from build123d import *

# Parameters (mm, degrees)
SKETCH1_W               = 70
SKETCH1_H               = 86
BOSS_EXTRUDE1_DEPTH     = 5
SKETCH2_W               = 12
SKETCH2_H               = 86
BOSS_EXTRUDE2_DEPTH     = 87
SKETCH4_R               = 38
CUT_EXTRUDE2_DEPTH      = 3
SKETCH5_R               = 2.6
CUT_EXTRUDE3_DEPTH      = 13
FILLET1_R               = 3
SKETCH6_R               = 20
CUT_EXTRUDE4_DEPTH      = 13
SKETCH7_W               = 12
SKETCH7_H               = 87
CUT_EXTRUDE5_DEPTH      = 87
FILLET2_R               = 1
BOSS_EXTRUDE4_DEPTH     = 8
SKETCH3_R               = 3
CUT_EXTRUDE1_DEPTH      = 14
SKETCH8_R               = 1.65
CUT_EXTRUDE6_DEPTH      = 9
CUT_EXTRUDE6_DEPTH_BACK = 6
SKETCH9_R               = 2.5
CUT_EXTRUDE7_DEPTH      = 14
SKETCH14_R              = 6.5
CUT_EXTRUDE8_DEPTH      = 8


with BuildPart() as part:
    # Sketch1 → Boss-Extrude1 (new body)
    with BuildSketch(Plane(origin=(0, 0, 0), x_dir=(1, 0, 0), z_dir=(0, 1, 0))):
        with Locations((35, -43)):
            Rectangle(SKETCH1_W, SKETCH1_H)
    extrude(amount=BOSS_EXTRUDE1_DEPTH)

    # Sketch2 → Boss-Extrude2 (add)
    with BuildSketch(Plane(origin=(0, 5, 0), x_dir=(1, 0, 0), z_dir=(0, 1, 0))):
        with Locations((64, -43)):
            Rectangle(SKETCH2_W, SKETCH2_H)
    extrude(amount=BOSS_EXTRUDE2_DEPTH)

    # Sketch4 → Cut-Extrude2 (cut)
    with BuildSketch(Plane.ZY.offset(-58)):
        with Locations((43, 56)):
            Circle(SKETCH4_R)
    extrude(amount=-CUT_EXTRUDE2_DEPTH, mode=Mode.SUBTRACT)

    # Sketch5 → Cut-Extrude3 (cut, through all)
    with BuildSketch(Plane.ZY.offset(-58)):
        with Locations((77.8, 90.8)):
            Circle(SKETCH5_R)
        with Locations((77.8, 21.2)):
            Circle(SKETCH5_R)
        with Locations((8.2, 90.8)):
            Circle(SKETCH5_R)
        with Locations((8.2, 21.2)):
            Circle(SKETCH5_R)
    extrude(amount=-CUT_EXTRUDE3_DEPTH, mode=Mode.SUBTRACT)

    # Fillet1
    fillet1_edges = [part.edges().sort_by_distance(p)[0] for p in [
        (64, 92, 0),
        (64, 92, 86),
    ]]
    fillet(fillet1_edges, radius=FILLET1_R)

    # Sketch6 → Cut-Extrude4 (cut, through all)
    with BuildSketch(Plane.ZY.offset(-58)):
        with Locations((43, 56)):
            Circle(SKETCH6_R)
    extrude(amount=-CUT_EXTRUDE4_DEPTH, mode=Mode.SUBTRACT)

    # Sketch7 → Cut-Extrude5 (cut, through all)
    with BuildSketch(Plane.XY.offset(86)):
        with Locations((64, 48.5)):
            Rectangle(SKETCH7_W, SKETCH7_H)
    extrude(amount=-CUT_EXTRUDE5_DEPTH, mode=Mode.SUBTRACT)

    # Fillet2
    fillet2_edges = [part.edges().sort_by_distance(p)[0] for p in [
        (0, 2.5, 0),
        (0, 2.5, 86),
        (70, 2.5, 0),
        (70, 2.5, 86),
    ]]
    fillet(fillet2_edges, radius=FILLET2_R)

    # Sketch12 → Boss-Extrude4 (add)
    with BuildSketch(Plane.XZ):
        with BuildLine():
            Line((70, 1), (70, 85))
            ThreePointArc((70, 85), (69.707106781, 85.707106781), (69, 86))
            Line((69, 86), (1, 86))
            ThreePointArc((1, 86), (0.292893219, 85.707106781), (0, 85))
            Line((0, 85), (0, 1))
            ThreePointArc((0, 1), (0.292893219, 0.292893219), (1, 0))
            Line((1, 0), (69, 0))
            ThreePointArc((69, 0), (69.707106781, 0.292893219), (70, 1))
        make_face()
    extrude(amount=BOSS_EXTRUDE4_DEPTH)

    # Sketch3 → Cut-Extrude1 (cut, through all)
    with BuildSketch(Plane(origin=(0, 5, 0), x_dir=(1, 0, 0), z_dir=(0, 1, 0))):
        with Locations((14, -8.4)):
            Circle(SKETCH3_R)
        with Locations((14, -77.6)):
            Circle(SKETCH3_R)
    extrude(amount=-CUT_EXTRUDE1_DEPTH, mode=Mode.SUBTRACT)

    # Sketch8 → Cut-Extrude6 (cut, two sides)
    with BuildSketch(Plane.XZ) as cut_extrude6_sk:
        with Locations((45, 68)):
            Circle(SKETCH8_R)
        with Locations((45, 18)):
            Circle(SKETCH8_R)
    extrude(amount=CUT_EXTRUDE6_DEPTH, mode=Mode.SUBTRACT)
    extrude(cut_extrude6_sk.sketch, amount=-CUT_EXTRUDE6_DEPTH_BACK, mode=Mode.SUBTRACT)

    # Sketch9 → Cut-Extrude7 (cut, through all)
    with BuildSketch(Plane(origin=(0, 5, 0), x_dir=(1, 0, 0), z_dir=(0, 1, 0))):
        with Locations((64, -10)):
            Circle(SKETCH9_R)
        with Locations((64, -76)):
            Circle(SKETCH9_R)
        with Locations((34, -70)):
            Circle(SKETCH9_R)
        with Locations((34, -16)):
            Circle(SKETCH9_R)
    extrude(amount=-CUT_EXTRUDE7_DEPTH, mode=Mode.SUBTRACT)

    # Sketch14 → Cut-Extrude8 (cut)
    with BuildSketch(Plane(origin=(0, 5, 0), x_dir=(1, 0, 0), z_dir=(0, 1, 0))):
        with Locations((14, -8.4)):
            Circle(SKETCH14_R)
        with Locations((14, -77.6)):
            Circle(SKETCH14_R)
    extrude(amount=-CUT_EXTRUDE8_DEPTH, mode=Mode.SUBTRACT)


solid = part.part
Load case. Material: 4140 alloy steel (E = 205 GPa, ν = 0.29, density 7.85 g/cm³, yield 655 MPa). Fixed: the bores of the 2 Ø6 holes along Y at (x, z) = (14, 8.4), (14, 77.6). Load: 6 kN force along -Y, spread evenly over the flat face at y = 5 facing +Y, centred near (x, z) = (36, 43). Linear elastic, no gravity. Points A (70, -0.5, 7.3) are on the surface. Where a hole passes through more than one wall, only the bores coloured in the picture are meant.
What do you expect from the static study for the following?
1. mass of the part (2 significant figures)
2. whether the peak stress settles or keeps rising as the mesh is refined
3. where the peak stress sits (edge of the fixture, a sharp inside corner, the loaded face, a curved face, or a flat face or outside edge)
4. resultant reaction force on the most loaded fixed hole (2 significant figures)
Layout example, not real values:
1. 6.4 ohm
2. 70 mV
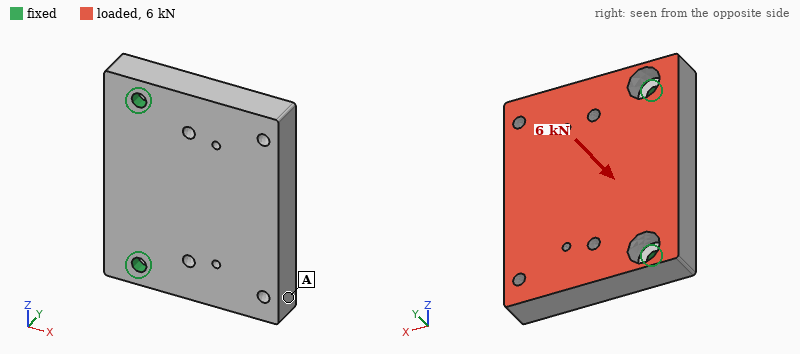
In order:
1. 590 g
2. keeps rising
3. edge of the fixture
4. 3.3 kN
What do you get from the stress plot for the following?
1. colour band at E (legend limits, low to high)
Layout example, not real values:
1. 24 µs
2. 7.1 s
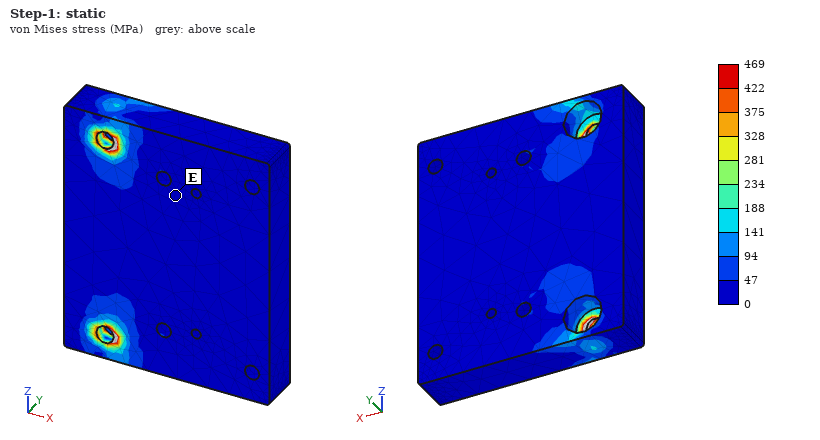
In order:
1. 0 to 47 MPa
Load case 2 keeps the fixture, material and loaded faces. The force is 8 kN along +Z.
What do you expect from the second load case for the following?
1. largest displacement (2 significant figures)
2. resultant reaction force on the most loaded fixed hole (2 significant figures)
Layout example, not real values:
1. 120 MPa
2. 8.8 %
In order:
1. 10 µm
2. 4.8 kN
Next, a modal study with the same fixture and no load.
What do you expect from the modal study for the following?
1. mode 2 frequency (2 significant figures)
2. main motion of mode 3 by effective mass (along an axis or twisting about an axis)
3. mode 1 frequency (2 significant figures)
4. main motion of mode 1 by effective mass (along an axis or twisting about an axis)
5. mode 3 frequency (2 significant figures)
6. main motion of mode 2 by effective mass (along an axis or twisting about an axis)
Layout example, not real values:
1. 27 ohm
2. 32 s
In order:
1. 4600 Hz
2. along Y
3. 1400 Hz
4. along Y
5. 8000 Hz
6. twisting about X
